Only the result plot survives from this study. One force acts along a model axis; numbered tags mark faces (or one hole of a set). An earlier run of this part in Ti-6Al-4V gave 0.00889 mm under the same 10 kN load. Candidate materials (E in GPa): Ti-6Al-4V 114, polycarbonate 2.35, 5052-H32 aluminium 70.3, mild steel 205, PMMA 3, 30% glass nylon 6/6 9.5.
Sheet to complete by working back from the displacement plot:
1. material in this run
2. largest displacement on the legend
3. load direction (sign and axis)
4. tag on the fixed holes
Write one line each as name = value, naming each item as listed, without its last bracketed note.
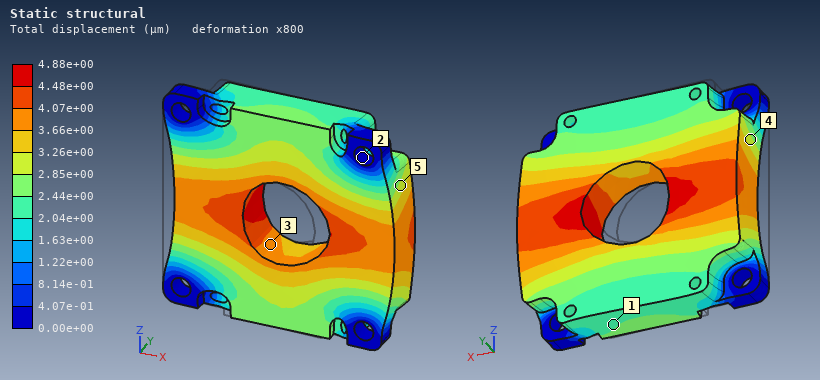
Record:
material in this run = mild steel
largest displacement on the legend = 4.88e+00 µm
load direction = +X
tag on the fixed holes = 2
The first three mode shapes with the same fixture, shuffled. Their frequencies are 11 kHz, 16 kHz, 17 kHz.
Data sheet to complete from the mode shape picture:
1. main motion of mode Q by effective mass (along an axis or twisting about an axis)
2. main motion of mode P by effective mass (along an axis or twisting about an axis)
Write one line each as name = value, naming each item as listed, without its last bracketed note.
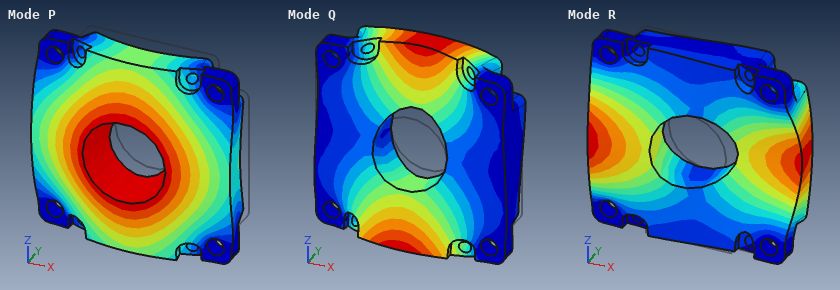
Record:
main motion of mode Q by effective mass = twisting about X
main motion of mode P by effective mass = along Y
